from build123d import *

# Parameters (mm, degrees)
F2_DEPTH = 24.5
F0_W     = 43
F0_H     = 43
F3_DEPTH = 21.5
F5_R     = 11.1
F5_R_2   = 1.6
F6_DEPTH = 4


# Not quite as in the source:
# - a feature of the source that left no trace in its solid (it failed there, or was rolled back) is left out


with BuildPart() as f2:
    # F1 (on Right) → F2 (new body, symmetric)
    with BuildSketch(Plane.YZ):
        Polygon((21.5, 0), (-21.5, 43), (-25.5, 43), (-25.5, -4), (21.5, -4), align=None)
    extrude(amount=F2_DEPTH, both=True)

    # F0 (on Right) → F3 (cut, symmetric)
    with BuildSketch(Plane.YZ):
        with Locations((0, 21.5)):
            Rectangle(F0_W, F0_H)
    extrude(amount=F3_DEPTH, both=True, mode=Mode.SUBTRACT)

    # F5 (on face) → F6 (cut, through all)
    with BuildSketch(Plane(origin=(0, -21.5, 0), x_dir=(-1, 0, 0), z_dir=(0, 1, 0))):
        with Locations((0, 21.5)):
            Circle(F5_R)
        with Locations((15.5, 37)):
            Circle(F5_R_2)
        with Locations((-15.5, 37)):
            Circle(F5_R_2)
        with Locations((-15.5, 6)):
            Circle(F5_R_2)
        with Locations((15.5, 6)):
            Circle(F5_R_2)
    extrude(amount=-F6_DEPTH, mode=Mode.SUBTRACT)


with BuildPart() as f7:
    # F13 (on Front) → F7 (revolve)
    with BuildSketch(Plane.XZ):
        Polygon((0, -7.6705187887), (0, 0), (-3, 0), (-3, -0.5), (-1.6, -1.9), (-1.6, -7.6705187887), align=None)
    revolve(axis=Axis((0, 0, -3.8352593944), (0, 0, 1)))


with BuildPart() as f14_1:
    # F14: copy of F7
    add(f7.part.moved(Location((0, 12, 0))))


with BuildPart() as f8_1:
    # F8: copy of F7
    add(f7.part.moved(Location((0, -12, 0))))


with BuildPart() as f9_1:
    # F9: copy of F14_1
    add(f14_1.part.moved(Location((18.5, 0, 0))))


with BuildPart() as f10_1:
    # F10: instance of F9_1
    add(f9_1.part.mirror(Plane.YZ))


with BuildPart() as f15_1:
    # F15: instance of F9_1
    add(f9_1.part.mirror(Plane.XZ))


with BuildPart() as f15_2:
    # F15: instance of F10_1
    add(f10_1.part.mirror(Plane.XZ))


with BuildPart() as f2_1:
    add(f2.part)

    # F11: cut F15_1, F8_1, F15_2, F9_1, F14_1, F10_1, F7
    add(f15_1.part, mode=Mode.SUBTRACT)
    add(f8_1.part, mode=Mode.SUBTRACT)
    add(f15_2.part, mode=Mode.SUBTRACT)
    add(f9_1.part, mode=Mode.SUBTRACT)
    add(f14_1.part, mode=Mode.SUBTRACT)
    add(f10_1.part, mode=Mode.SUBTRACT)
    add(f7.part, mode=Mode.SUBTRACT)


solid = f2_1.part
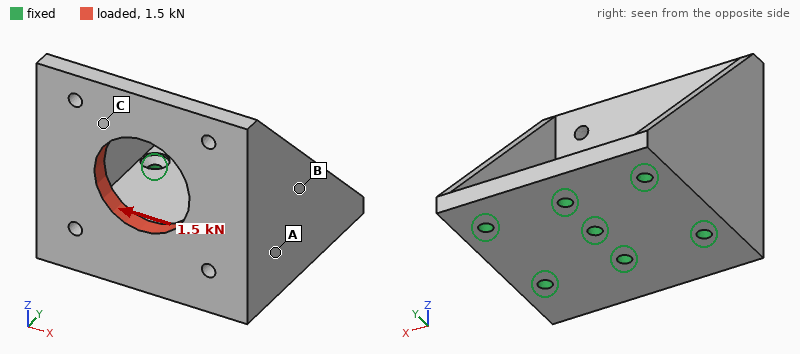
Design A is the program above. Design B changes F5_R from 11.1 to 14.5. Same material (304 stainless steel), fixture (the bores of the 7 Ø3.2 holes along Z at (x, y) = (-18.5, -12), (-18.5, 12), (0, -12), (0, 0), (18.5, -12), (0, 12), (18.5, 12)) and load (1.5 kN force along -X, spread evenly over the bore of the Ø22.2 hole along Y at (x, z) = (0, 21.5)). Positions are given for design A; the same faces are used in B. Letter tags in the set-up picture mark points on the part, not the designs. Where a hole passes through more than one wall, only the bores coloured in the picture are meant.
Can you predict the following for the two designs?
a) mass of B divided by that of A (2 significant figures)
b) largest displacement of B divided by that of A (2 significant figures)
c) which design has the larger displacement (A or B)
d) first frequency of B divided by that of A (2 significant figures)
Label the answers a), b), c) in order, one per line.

a) 0.95
b) 1.2
c) B
d) 0.99
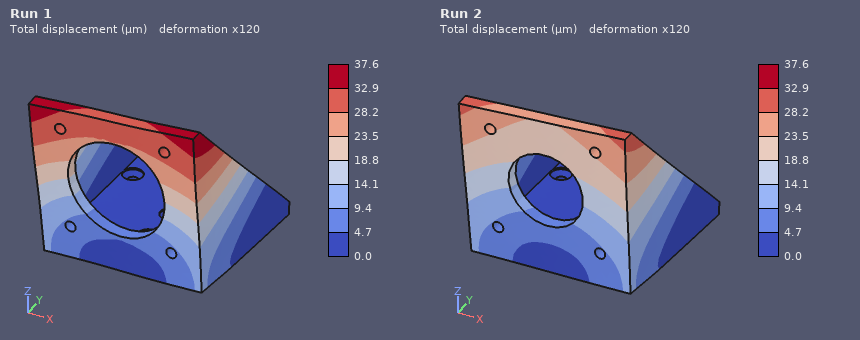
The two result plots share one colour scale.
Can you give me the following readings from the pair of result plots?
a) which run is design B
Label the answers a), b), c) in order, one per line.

a) Run 1
